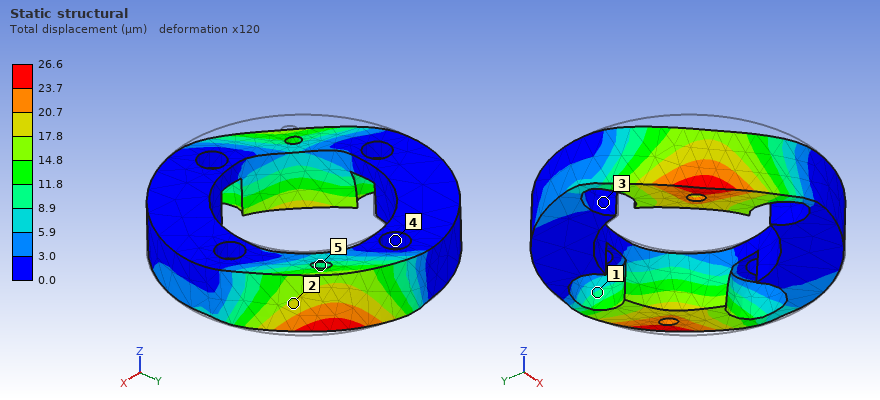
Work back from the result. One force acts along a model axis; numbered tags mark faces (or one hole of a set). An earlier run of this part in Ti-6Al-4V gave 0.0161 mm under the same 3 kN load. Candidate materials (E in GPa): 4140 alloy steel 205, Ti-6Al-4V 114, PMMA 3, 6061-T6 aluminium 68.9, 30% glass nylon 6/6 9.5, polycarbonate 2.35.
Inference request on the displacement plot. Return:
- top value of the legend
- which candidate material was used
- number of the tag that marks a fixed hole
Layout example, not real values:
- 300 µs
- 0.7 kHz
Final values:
- 26.6 µm
- 6061-T6 aluminium
- 4
